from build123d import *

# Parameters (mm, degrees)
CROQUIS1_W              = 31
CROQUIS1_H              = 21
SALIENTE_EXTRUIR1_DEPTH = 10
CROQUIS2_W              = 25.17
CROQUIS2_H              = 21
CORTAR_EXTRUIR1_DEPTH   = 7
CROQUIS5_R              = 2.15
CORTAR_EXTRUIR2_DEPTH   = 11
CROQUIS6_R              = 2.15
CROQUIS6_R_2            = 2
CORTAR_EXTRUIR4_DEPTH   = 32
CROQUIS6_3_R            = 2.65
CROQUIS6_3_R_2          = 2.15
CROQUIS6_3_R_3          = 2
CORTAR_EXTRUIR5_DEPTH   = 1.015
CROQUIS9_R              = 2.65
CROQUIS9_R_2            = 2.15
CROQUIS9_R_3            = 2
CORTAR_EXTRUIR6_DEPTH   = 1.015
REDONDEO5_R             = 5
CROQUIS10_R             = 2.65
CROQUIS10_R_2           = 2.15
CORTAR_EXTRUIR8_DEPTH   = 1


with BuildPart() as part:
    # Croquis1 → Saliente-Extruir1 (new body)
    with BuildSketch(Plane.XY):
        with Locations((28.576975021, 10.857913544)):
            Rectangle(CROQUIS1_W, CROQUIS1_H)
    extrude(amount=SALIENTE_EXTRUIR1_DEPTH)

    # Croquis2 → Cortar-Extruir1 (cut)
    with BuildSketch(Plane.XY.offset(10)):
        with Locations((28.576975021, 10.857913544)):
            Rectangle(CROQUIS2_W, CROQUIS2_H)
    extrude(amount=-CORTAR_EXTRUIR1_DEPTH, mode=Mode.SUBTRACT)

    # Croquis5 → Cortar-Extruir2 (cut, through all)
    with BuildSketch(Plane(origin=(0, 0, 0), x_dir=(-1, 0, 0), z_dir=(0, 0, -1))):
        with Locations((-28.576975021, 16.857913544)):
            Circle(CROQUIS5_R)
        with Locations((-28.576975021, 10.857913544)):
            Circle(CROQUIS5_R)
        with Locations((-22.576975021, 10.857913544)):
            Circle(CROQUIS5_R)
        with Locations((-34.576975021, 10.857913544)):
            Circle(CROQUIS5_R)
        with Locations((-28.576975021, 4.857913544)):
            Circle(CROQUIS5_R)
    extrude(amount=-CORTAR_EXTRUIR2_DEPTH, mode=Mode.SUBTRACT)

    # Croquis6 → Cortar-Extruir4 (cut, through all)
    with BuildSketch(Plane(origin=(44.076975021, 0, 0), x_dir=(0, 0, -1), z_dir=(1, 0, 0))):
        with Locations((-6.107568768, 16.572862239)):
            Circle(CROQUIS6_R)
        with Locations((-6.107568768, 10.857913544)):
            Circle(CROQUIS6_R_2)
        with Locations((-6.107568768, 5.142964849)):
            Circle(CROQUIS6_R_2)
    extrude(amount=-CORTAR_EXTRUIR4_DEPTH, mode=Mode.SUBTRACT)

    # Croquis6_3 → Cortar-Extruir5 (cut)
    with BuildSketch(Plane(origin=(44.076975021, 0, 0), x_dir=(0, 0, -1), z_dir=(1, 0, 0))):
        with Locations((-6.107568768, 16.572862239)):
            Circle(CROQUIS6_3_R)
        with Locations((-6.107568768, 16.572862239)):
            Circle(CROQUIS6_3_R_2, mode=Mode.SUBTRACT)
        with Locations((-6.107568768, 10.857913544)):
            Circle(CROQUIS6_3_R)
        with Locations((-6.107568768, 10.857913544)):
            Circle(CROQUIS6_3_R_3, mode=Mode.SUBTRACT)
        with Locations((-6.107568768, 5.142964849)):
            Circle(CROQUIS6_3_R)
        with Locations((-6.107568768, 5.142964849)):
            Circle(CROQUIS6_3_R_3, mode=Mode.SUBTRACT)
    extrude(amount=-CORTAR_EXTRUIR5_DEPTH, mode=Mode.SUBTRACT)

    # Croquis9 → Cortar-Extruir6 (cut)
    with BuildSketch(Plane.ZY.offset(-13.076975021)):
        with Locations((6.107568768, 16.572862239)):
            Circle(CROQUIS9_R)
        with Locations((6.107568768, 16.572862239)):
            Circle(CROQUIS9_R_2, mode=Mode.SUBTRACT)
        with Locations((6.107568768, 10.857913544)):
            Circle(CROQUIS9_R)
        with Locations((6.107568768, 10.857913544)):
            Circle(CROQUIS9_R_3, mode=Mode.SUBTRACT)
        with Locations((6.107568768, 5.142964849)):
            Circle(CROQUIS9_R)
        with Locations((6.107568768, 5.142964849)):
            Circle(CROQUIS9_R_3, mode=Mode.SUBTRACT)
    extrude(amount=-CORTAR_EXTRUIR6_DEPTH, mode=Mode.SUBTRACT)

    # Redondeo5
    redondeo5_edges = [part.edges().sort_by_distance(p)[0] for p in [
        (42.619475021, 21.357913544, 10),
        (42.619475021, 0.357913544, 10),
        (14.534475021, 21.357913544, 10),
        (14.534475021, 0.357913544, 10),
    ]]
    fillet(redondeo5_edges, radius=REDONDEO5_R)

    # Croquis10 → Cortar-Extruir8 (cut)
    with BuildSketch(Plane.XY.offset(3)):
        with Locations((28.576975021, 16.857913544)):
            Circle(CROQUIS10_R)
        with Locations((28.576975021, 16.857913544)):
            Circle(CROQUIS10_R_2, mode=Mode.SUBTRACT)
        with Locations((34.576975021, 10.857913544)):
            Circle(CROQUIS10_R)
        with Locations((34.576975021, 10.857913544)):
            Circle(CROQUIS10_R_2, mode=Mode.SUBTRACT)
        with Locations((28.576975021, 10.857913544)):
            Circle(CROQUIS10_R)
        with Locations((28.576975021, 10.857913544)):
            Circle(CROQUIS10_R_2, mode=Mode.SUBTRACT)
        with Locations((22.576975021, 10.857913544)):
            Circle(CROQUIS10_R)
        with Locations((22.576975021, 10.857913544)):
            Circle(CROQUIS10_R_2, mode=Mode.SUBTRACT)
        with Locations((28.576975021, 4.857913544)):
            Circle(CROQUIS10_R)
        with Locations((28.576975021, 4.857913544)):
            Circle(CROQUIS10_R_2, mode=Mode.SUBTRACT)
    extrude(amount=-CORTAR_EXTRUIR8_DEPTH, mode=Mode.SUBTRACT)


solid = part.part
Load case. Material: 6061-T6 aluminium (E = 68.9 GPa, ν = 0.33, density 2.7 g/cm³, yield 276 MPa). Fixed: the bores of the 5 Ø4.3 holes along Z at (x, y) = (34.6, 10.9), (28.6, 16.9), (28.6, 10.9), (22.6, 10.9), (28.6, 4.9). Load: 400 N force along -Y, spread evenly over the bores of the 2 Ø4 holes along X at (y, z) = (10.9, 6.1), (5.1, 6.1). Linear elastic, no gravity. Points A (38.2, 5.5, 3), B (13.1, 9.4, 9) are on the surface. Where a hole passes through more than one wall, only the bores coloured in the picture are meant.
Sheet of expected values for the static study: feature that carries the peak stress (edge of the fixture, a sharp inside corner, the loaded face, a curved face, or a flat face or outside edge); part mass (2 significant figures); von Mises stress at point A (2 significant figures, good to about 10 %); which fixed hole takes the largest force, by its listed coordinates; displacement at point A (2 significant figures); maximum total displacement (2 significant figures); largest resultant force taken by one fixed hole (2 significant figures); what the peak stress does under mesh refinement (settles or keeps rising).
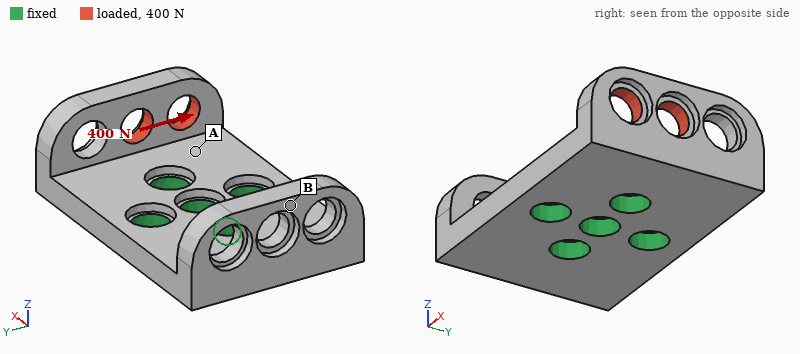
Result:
edge of the fixture
6.0 g
41 MPa
(34.6, 10.9)
9.7 µm
38 µm
360 N
keeps rising
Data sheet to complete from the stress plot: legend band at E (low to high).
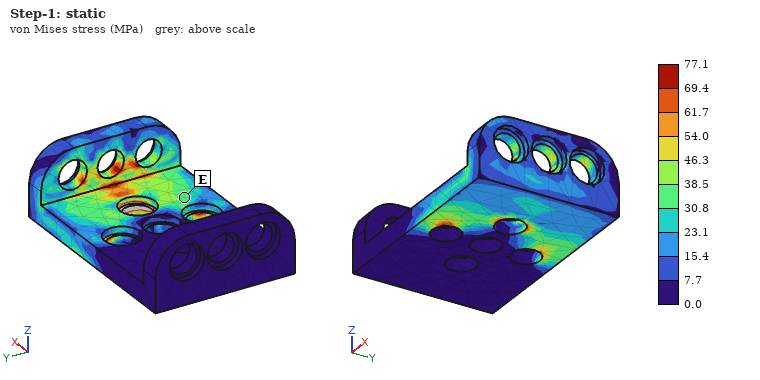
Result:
30.8 to 38.5 MPa
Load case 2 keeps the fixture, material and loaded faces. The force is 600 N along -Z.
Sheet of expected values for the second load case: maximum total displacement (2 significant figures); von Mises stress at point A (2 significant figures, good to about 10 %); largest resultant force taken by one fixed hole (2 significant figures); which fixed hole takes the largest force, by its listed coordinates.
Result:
92 µm
70 MPa
860 N
(34.6, 10.9)
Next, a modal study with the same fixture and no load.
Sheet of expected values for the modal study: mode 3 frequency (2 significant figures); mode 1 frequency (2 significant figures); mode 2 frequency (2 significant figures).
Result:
14 kHz
13 kHz
13 kHz
